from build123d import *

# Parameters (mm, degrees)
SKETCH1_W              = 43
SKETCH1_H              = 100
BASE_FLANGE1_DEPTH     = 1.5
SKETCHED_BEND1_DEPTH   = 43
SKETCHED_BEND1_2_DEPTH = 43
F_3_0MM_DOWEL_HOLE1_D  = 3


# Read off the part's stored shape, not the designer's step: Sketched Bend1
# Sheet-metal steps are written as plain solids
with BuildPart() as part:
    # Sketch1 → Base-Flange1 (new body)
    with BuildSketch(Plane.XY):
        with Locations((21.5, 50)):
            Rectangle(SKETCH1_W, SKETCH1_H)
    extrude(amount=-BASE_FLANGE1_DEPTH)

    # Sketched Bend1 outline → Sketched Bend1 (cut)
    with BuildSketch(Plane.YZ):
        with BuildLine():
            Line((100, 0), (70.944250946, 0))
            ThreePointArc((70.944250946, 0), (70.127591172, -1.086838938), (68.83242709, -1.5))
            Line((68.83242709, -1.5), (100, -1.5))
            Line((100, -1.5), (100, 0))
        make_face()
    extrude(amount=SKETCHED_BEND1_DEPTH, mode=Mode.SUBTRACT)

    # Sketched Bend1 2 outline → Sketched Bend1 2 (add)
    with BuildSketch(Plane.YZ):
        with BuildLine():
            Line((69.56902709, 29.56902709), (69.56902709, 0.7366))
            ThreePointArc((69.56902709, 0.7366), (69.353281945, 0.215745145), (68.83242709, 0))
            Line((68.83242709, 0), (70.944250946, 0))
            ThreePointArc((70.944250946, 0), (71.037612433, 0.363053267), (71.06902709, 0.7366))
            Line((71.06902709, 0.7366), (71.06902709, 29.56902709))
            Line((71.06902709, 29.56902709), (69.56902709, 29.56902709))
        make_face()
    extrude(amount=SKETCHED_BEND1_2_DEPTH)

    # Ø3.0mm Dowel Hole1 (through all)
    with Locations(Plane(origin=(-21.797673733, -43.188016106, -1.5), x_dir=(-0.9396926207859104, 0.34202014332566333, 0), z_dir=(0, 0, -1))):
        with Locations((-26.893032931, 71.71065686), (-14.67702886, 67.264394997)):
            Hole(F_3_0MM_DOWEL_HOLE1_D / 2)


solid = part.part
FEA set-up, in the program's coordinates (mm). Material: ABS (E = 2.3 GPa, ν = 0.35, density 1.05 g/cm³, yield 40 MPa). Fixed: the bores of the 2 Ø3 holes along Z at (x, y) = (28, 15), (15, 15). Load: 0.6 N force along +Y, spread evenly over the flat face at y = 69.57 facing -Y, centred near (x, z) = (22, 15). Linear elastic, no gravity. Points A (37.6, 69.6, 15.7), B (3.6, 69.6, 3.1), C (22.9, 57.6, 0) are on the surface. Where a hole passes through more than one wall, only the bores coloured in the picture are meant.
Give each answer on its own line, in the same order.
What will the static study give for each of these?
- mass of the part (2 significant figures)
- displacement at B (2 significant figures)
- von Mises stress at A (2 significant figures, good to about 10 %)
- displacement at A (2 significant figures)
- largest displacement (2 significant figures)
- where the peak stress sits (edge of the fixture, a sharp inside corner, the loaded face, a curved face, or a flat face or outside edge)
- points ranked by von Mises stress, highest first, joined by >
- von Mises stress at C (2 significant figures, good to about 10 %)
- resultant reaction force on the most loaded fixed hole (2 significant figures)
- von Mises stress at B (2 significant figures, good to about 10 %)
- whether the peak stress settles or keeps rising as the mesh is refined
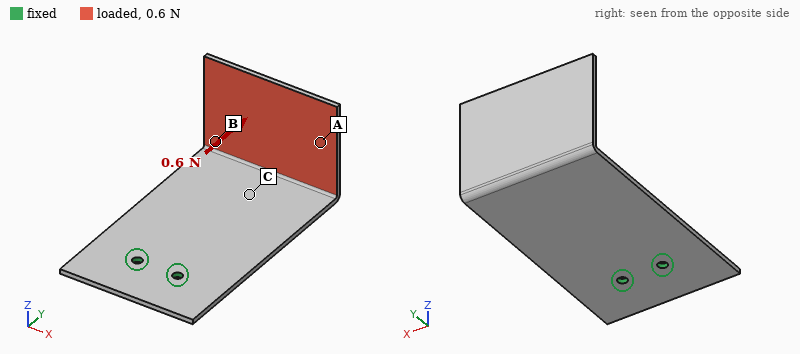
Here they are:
6.8 g
0.50 mm
0.12 MPa
0.59 mm
0.81 mm
edge of the fixture
C > B > A
0.54 MPa
0.30 N
0.35 MPa
keeps rising
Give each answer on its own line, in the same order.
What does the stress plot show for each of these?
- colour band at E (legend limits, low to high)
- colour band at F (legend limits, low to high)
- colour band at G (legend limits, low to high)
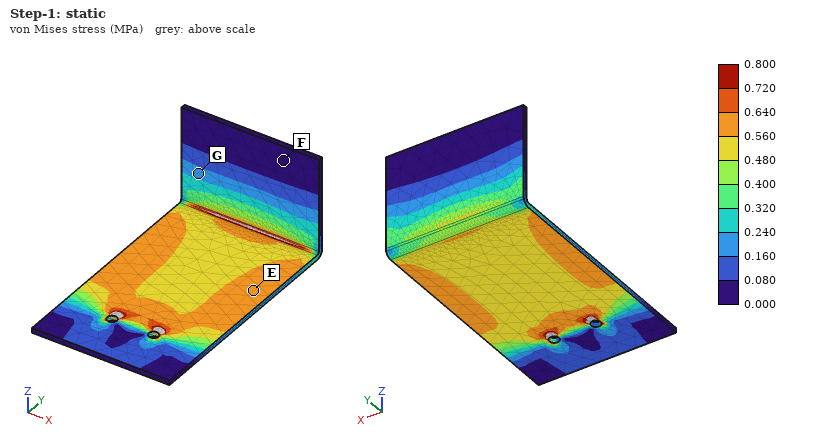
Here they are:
0.560 to 0.640 MPa
0.000 to 0.080 MPa
0.160 to 0.240 MPa
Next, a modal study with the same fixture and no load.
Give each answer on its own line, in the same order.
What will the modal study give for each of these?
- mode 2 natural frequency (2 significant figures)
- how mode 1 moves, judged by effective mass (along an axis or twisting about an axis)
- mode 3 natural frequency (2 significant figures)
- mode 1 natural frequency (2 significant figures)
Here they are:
140 Hz
along Z
240 Hz
62 Hz
